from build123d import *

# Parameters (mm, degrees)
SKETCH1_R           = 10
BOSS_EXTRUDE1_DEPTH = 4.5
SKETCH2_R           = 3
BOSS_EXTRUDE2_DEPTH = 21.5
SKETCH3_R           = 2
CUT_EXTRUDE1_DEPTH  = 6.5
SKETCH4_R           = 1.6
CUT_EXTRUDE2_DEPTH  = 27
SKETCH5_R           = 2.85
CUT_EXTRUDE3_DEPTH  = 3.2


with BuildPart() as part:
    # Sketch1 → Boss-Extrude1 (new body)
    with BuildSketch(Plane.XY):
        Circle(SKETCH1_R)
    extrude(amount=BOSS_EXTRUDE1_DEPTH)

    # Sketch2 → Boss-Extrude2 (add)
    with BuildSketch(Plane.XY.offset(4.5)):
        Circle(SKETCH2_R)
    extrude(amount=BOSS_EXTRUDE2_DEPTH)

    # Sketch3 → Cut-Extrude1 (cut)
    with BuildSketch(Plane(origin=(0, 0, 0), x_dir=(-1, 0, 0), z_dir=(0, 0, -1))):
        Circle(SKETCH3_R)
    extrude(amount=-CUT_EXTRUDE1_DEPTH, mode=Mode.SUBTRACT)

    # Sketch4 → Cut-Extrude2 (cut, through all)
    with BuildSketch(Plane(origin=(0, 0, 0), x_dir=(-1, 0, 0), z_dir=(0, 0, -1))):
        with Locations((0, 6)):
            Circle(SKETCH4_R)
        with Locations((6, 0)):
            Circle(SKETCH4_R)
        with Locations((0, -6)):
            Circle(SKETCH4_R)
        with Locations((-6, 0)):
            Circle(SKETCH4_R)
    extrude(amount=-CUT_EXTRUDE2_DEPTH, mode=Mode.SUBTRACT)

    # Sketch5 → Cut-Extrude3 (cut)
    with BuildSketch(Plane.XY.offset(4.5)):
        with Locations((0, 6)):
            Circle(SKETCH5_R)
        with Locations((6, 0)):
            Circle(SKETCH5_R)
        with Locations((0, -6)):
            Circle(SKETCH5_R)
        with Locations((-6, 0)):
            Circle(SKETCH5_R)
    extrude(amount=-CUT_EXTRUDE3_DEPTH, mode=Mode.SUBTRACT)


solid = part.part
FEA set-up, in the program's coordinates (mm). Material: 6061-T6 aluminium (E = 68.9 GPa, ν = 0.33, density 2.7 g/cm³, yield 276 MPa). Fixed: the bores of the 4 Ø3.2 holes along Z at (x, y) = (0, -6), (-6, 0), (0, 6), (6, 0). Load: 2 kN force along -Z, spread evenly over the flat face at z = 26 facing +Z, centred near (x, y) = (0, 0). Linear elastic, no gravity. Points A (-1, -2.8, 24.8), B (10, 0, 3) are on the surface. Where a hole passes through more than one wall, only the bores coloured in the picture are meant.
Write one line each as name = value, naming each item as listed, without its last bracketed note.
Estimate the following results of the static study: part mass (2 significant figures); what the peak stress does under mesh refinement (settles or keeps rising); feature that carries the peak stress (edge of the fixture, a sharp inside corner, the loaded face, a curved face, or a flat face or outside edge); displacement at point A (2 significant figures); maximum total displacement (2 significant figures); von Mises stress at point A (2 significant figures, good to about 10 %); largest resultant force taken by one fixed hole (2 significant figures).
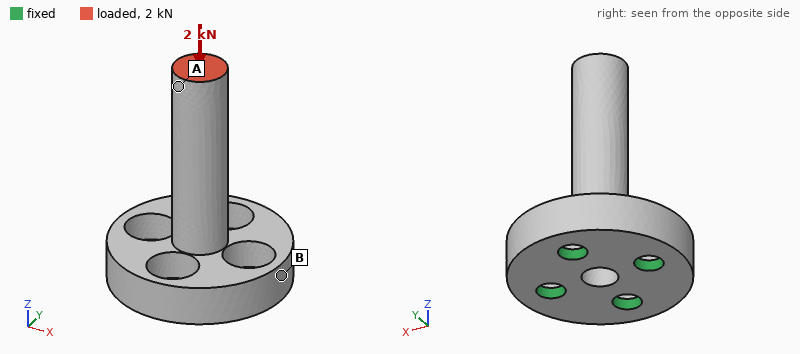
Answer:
part mass = 4.2 g
what the peak stress does under mesh refinement = keeps rising
feature that carries the peak stress = edge of the fixture
displacement at point A = 33 µm
maximum total displacement = 34 µm
von Mises stress at point A = 71 MPa
largest resultant force taken by one fixed hole = 560 N
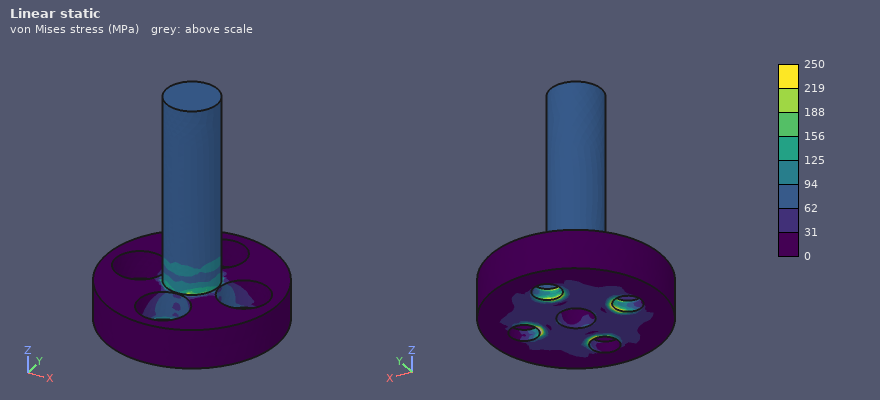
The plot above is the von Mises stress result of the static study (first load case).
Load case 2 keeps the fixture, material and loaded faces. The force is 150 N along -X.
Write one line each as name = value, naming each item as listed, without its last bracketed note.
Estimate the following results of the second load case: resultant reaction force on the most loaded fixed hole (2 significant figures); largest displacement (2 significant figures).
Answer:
resultant reaction force on the most loaded fixed hole = 320 N
largest displacement = 0.18 mm
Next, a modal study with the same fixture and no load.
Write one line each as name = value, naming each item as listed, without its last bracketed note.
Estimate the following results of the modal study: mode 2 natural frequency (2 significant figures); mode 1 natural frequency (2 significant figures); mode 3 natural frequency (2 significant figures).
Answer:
mode 2 natural frequency = 6700 Hz
mode 1 natural frequency = 6700 Hz
mode 3 natural frequency = 33 kHz
